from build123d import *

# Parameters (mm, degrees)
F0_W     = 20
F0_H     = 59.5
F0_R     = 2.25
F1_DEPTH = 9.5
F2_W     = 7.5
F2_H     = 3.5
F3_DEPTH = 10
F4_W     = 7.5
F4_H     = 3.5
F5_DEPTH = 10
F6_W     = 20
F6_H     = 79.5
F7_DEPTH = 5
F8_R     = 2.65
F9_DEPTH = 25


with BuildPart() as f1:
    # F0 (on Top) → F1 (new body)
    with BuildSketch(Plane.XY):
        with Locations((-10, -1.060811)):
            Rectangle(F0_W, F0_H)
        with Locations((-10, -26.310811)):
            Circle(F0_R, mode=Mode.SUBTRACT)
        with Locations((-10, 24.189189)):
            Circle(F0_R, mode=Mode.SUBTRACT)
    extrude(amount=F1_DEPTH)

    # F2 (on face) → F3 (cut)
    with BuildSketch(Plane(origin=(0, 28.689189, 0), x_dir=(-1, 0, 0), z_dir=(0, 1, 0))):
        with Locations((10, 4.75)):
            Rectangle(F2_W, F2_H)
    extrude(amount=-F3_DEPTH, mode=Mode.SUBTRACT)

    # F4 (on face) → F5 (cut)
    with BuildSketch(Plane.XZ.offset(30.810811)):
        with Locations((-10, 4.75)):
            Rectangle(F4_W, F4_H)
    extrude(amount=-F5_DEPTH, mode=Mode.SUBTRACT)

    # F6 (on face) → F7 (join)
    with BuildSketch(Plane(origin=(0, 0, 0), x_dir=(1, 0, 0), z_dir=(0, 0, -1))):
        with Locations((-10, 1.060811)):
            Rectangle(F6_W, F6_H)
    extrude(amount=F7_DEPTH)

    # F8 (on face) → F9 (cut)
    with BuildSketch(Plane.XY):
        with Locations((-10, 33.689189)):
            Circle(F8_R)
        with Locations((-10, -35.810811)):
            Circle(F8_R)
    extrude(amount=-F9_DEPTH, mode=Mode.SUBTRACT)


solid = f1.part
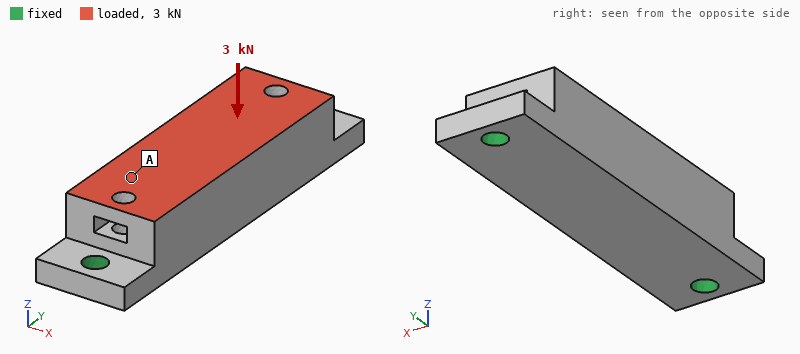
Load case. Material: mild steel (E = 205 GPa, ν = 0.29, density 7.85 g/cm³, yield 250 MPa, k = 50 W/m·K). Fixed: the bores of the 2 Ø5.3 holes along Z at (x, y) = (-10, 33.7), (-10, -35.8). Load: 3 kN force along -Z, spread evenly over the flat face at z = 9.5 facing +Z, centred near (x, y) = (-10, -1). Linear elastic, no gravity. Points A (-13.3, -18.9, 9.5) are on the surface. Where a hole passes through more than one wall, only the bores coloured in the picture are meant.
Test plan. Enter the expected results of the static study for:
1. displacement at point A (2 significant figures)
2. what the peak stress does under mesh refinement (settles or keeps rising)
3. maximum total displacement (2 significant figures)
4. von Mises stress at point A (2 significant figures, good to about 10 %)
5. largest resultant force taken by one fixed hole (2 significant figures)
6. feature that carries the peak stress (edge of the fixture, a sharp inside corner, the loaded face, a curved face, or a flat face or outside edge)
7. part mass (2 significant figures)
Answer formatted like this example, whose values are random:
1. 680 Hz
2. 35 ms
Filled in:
1. 7.1 µm
2. keeps rising
3. 9.6 µm
4. 14 MPa
5. 2.0 kN
6. edge of the fixture
7. 140 g
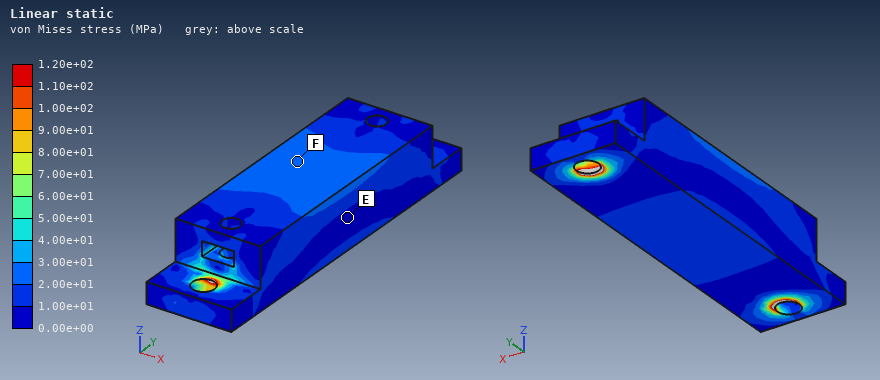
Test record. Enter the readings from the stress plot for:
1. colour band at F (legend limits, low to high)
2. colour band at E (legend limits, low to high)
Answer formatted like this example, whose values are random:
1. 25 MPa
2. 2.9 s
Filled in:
1. 2.00e+01 to 3.00e+01 MPa
2. 0.00e+00 to 1.00e+01 MPa
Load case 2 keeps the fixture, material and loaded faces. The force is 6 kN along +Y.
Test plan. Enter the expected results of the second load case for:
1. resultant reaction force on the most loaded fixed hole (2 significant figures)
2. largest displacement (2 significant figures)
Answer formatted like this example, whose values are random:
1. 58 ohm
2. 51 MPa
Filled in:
1. 3.2 kN
2. 5.2 µm
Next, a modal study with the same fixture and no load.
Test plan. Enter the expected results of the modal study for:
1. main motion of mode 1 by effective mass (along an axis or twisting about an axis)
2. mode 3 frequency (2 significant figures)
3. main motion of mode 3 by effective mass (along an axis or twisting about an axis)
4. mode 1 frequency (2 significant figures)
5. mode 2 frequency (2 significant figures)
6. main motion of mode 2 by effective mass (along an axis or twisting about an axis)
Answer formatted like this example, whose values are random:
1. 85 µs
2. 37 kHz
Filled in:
1. along X
2. 12 kHz
3. along X
4. 6600 Hz
5. 8500 Hz
6. along Z
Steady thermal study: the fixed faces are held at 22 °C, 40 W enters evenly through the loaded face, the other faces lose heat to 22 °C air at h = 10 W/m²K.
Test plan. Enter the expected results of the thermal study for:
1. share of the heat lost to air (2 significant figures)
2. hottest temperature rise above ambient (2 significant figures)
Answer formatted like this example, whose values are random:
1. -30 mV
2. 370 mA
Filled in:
1. 4.4 %
2. 56 K
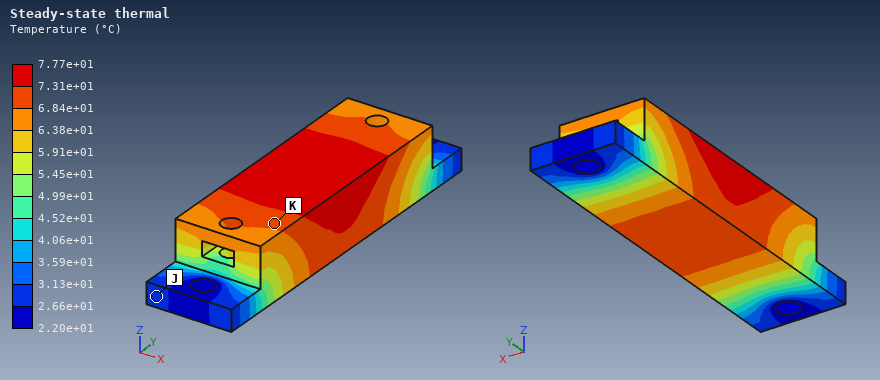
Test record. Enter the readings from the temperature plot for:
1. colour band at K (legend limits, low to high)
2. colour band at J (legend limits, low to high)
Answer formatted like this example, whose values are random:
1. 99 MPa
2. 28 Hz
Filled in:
1. 6.84e+01 to 7.31e+01 °C
2. 2.66e+01 to 3.13e+01 °C
